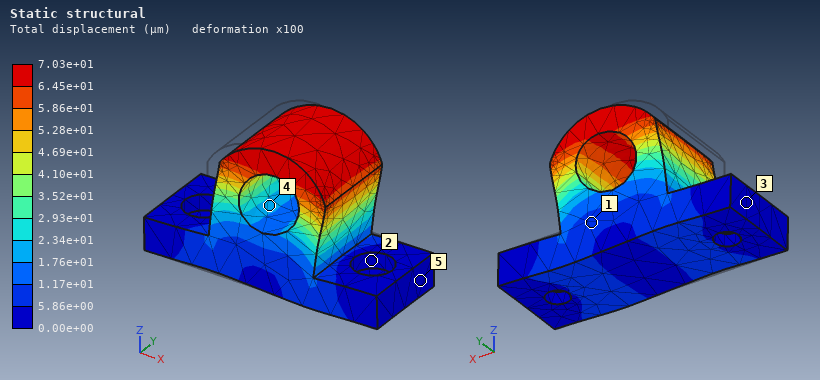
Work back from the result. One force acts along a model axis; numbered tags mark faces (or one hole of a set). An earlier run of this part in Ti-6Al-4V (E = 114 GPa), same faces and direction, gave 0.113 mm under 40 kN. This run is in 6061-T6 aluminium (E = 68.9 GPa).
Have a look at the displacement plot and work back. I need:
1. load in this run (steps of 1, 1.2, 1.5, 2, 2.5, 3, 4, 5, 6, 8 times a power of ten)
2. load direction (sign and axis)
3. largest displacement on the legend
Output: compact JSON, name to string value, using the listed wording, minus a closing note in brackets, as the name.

{"load in this run": "15 kN", "load direction": "+X", "largest displacement on the legend": "7.03e+01 µm"}
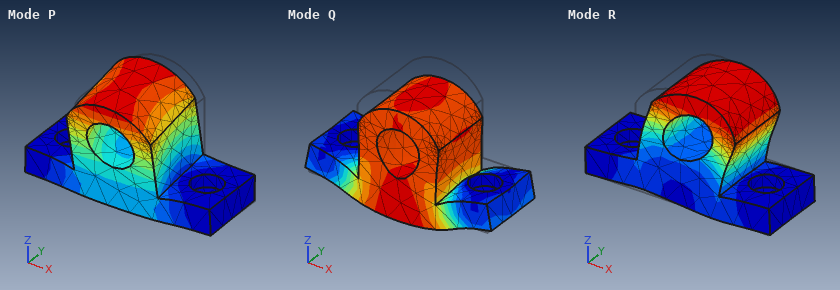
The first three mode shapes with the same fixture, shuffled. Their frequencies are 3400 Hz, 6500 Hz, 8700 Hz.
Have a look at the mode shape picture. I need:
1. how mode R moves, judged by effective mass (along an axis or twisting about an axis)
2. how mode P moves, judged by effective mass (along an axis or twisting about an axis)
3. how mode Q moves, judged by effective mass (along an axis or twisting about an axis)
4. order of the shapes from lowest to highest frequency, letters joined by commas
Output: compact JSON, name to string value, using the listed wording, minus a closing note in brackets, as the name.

{"how mode R moves, judged by effective mass": "along X", "how mode P moves, judged by effective mass": "along Y", "how mode Q moves, judged by effective mass": "along Z", "order of the shapes from lowest to highest frequency, letters joined by commas": "P, R, Q"}
